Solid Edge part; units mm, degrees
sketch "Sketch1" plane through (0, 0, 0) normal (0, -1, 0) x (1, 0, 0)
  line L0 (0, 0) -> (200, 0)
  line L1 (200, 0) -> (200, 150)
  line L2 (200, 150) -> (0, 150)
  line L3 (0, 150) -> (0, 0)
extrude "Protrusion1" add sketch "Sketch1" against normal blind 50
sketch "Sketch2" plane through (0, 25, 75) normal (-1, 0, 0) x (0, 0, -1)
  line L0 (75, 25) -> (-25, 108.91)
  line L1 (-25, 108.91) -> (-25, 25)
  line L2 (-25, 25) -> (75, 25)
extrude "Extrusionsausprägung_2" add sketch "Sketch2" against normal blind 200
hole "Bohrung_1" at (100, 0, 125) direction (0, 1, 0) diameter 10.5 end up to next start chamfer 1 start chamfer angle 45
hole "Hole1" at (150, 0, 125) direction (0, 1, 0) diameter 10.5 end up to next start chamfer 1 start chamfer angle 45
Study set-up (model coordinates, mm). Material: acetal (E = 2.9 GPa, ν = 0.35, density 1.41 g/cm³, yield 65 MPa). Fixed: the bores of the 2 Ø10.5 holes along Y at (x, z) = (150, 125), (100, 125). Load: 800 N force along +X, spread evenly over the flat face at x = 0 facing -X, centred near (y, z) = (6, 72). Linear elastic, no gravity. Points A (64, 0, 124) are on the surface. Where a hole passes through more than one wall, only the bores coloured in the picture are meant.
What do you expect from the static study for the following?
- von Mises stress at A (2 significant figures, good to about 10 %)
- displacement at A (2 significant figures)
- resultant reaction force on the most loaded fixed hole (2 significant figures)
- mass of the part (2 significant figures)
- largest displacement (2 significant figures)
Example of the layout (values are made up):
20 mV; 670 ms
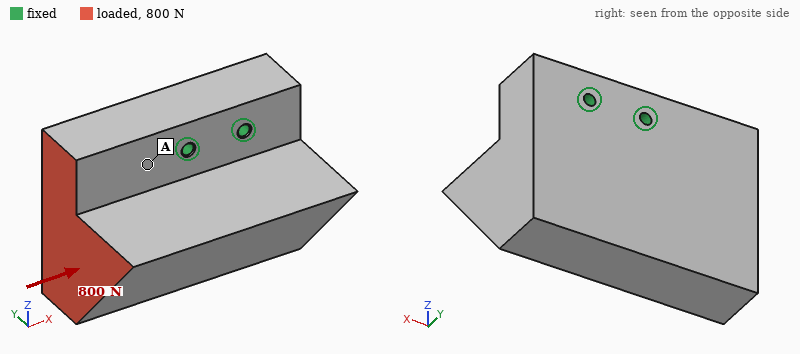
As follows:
0.19 MPa; 10 µm; 880 N; 3.3 kg; 42 µm
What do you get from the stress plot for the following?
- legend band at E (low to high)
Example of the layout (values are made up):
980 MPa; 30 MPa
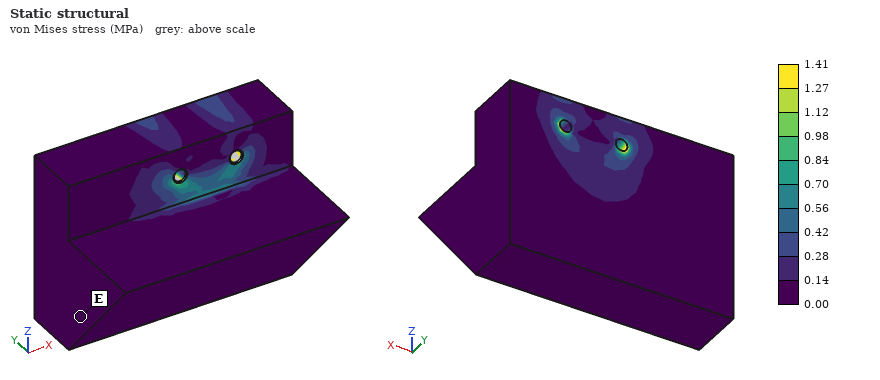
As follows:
0.00 to 0.14 MPa
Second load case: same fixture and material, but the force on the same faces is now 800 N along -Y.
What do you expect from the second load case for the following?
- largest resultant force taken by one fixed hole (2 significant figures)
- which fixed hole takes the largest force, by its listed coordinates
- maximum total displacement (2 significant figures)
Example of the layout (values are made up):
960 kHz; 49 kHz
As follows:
1.3 kN; (100, 125); 0.16 mm
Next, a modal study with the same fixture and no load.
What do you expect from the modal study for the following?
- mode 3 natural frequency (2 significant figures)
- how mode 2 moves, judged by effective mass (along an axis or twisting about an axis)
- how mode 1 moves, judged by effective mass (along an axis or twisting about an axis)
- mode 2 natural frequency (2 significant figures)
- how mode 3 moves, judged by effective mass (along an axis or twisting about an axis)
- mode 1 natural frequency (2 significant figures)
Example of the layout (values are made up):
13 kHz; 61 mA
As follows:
540 Hz; along X; along Y; 440 Hz; twisting about Z; 340 Hz
